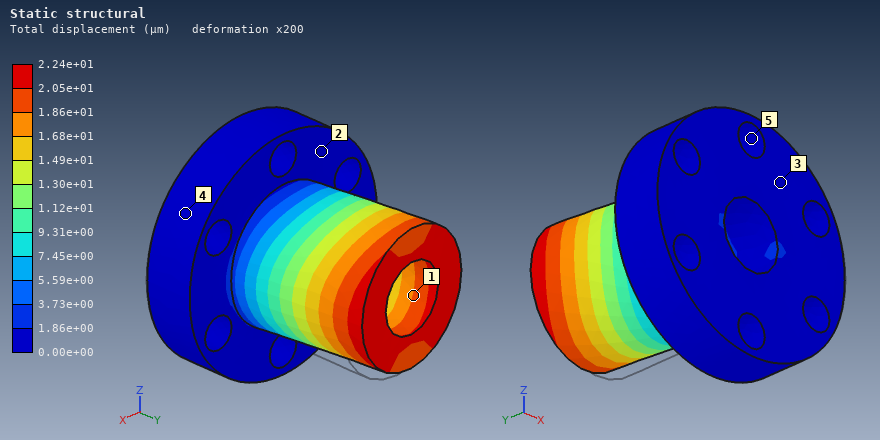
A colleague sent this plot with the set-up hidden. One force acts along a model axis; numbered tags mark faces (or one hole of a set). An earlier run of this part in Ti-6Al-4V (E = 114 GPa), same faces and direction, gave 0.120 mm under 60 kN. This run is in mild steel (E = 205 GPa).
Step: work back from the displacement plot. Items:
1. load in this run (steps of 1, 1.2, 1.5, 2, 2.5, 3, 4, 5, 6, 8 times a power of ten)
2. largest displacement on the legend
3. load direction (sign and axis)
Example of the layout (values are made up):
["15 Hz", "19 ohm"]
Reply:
["20 kN", "2.24e+01 µm", "-X"]
